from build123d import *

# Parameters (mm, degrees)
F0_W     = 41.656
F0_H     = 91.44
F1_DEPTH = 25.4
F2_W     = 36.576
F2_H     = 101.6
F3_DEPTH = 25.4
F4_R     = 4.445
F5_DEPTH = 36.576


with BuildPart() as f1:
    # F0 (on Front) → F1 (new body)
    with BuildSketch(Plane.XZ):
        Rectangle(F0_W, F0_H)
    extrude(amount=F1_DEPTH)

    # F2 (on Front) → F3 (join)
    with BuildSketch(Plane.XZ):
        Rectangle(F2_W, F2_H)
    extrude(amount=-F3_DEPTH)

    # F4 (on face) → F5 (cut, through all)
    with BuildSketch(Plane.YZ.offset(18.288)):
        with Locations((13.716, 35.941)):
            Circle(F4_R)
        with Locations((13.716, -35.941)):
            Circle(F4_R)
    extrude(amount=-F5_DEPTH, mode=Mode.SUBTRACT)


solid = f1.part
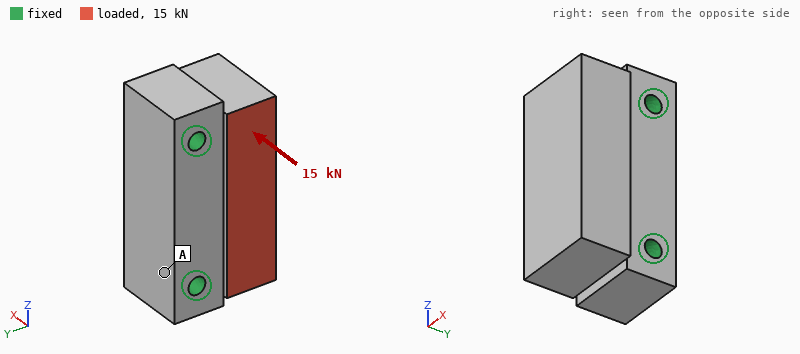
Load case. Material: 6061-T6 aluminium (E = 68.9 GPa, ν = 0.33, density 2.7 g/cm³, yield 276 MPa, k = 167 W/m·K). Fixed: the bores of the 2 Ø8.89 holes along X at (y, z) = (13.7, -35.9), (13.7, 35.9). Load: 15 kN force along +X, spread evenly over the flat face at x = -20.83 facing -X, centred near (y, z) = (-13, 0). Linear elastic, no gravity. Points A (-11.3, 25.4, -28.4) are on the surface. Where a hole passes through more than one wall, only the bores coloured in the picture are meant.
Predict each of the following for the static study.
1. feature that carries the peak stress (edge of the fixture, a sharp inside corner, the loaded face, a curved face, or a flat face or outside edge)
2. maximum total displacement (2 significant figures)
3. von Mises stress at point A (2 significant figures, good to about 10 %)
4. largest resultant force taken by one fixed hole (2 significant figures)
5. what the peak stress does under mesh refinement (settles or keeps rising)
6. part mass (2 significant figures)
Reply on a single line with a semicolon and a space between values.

edge of the fixture; 25 µm; 7.4 MPa; 7.5 kN; keeps rising; 500 g
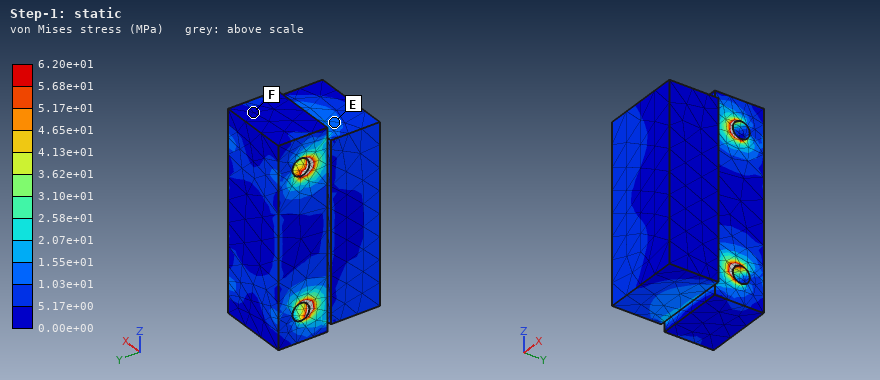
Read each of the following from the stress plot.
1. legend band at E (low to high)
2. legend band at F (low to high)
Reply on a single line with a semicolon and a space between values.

1.03e+01 to 1.55e+01 MPa; 0.00e+00 to 5.17e+00 MPa
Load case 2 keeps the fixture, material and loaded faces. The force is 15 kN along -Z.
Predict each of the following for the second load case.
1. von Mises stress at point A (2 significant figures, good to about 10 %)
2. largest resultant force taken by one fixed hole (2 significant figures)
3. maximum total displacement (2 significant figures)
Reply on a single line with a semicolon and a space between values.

3.5 MPa; 9.6 kN; 17 µm
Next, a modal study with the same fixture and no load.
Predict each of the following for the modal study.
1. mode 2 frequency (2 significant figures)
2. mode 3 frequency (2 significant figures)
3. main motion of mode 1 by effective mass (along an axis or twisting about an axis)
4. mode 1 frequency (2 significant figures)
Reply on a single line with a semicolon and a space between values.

15 kHz; 15 kHz; along X; 9100 Hz
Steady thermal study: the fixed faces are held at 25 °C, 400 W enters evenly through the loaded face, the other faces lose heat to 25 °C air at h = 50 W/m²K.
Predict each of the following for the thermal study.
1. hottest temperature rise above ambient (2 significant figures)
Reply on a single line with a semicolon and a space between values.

37 K
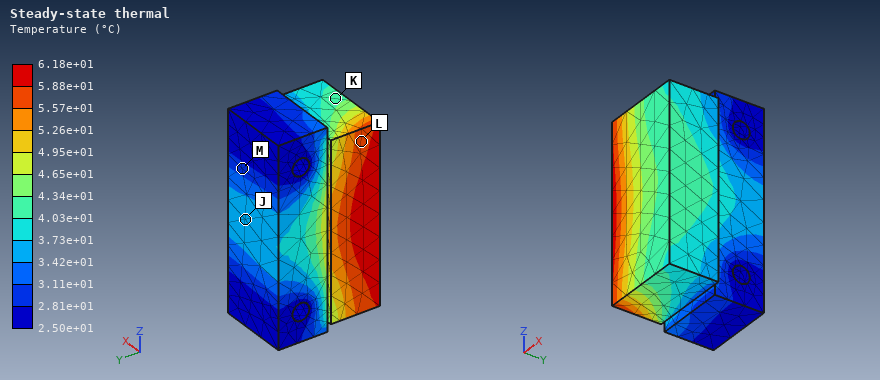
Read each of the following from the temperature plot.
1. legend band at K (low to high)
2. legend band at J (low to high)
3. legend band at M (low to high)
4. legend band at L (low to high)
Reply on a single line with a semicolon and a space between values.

4.03e+01 to 4.34e+01 °C; 3.42e+01 to 3.73e+01 °C; 2.81e+01 to 3.11e+01 °C; 5.57e+01 to 5.88e+01 °C
